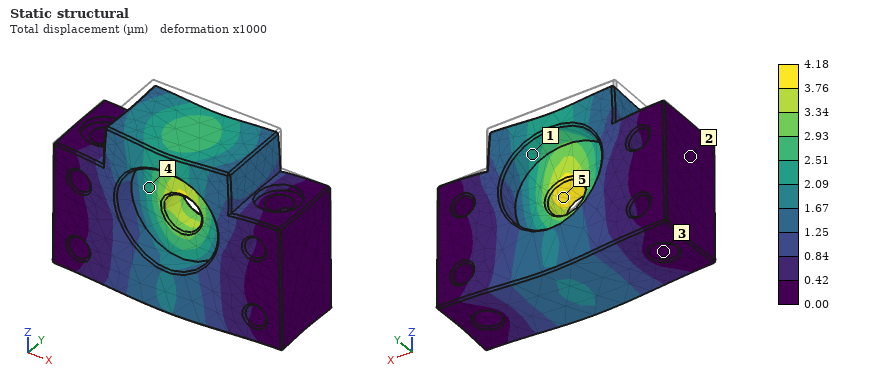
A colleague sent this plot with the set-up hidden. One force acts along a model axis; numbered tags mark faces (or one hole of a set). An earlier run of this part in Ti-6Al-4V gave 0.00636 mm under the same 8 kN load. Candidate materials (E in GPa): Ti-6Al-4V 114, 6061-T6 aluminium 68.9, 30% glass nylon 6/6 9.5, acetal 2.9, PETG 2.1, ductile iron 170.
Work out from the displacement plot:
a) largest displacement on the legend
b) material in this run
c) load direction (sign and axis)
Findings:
4.18 µm
ductile iron
-Z
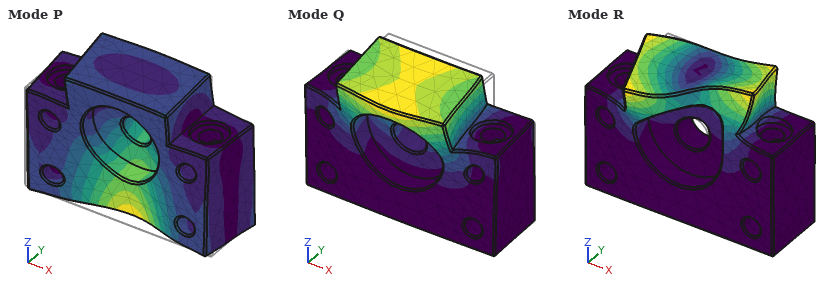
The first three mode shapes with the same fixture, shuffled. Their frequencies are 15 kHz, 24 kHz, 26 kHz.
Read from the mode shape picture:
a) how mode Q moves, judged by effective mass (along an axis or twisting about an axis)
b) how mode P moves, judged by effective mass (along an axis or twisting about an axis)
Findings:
along Y
along Y
